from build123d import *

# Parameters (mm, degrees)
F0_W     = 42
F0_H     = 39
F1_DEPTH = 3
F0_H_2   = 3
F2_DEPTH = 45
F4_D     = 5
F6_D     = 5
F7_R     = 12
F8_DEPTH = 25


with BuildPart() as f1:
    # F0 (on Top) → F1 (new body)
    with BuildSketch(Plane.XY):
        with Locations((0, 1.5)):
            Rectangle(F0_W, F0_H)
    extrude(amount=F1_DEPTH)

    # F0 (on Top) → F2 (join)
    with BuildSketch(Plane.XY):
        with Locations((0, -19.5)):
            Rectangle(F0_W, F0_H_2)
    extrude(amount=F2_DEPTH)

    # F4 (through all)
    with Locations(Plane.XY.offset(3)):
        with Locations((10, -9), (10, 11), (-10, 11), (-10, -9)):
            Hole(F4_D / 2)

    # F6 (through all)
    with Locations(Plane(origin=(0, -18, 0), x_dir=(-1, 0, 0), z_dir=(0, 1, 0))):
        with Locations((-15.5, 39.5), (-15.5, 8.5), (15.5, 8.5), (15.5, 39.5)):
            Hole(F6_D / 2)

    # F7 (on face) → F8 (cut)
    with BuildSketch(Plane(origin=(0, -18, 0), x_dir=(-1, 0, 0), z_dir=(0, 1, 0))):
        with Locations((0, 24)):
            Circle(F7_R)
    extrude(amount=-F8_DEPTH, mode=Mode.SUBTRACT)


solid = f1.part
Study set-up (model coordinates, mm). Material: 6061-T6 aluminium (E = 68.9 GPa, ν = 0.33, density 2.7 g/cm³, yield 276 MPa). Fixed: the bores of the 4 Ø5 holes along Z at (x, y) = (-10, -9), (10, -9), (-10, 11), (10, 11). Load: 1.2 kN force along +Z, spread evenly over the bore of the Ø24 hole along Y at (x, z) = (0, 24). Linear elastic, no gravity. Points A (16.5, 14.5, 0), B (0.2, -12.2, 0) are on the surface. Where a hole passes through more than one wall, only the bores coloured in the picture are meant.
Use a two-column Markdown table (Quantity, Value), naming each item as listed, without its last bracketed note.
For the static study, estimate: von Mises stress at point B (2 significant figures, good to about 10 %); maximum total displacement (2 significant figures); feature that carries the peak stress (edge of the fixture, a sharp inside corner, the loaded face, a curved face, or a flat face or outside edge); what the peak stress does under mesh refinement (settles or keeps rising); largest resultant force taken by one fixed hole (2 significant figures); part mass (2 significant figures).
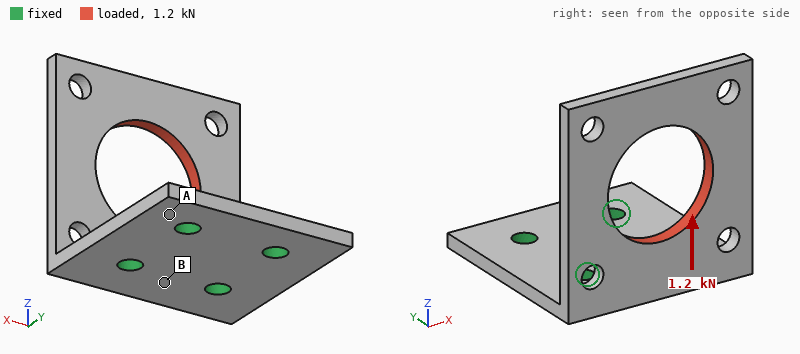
| Quantity | Value |
|---|---|
| von Mises stress at point B | 74 MPa |
| maximum total displacement | 0.37 mm |
| feature that carries the peak stress | edge of the fixture |
| what the peak stress does under mesh refinement | keeps rising |
| largest resultant force taken by one fixed hole | 650 N |
| part mass | 24 g |
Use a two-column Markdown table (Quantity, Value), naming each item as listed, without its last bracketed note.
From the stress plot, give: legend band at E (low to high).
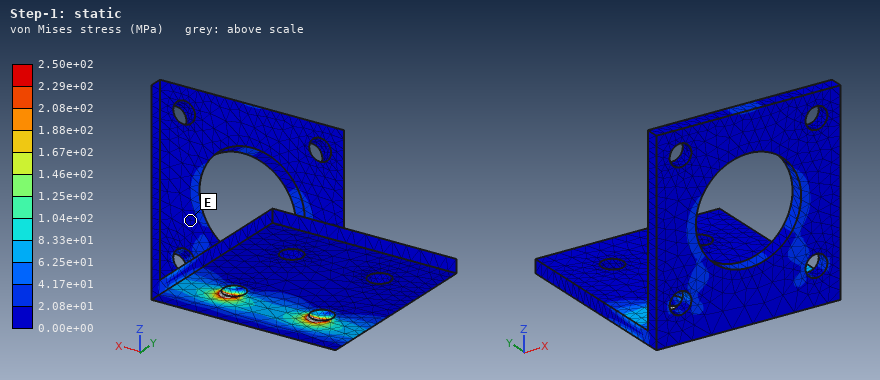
| Quantity | Value |
|---|---|
| legend band at E | 0.00e+00 to 2.08e+01 MPa |
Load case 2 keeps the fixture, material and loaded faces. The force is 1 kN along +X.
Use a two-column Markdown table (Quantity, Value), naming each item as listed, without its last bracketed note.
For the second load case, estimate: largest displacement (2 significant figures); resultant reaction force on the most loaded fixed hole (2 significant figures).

| Quantity | Value |
|---|---|
| largest displacement | 0.33 mm |
| resultant reaction force on the most loaded fixed hole | 1.1 kN |
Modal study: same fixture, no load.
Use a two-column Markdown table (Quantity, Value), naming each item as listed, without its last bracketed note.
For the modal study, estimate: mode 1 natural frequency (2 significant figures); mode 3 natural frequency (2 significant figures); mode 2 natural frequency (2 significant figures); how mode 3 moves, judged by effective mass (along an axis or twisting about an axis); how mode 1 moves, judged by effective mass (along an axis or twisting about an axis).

| Quantity | Value |
|---|---|
| mode 1 natural frequency | 960 Hz |
| mode 3 natural frequency | 3500 Hz |
| mode 2 natural frequency | 2400 Hz |
| how mode 3 moves, judged by effective mass | along X |
| how mode 1 moves, judged by effective mass | along Y |
